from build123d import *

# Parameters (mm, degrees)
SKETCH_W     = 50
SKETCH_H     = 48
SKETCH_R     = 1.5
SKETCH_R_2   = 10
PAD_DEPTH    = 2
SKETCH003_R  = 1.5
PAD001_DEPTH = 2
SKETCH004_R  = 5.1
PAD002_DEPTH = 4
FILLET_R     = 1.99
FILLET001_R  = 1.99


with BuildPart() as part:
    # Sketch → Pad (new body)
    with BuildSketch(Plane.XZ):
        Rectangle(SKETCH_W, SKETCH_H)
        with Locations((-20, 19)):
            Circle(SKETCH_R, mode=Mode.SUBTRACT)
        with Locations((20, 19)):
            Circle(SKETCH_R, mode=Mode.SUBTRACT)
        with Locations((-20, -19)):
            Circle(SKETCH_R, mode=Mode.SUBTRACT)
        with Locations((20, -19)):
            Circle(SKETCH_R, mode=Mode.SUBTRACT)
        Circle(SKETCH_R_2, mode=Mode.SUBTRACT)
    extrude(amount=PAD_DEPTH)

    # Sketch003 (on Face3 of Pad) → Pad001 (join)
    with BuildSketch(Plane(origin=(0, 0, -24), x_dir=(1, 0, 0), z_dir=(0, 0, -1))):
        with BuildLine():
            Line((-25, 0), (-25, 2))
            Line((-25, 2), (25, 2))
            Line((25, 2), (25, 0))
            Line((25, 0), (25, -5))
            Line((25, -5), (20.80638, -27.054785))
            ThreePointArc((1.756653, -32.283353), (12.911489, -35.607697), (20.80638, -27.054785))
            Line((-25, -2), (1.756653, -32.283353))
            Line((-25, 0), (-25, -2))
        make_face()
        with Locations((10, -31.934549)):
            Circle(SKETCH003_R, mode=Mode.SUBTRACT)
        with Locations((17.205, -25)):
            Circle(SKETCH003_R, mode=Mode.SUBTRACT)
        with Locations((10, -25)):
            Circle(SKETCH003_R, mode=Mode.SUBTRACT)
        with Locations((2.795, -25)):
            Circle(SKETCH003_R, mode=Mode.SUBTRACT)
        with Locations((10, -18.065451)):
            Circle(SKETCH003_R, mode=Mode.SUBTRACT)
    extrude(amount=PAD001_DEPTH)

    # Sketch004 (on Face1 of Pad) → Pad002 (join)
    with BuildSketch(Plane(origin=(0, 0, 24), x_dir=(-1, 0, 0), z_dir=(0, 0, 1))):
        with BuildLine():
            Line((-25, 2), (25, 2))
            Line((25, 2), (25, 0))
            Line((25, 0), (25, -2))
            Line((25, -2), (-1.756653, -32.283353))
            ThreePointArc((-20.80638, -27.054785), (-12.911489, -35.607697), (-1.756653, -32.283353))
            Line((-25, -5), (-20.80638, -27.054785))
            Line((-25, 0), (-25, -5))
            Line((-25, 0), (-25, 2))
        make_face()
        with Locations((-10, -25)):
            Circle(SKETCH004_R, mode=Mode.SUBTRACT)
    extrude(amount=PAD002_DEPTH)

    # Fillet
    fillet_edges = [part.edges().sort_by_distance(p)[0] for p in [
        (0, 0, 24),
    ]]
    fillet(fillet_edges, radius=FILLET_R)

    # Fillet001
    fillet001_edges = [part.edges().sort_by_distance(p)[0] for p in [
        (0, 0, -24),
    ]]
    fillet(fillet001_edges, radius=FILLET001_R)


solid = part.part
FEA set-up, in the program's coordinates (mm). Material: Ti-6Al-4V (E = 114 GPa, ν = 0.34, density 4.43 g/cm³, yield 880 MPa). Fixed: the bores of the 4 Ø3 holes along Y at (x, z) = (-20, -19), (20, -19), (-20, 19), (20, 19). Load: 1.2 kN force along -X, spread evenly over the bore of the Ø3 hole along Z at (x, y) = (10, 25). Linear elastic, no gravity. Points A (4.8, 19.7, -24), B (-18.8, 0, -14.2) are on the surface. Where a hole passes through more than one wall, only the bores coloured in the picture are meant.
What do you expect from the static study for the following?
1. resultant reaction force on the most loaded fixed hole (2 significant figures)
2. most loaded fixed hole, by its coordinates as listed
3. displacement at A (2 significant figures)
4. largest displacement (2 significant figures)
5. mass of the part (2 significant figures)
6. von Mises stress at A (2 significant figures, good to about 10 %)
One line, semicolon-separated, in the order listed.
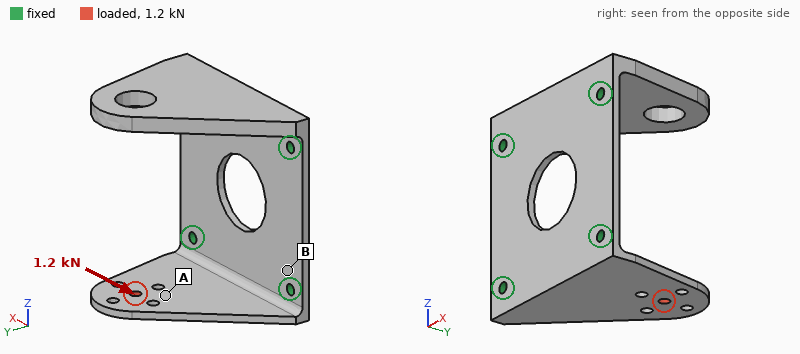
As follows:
1.1 kN; (-20, -19); 0.059 mm; 0.14 mm; 51 g; 56 MPa
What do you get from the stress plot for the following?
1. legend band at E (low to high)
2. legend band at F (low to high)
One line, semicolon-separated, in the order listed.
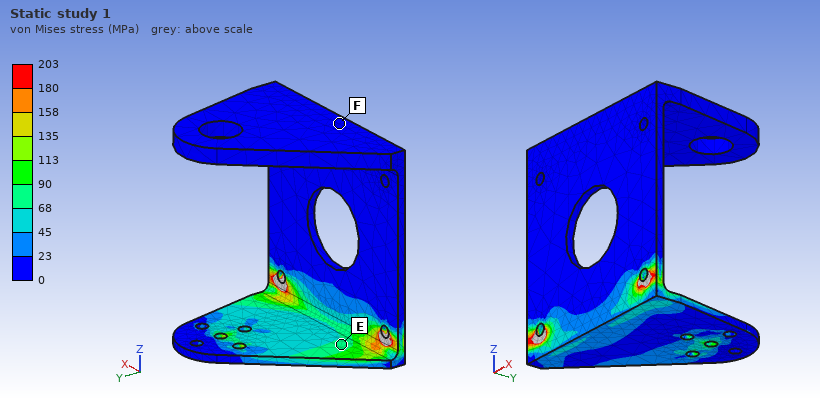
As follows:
68 to 90 MPa; 0 to 23 MPa
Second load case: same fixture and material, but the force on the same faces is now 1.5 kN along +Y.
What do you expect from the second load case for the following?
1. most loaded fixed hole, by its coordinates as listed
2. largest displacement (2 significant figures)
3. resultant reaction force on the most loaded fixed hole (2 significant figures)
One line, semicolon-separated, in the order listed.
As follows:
(20, -19); 0.34 mm; 1.2 kN
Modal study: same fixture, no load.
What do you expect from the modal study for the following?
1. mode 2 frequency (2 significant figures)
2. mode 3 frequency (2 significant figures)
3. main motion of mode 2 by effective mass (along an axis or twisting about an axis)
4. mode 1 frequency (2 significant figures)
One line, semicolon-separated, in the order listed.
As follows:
1500 Hz; 4700 Hz; along Z; 1400 Hz
